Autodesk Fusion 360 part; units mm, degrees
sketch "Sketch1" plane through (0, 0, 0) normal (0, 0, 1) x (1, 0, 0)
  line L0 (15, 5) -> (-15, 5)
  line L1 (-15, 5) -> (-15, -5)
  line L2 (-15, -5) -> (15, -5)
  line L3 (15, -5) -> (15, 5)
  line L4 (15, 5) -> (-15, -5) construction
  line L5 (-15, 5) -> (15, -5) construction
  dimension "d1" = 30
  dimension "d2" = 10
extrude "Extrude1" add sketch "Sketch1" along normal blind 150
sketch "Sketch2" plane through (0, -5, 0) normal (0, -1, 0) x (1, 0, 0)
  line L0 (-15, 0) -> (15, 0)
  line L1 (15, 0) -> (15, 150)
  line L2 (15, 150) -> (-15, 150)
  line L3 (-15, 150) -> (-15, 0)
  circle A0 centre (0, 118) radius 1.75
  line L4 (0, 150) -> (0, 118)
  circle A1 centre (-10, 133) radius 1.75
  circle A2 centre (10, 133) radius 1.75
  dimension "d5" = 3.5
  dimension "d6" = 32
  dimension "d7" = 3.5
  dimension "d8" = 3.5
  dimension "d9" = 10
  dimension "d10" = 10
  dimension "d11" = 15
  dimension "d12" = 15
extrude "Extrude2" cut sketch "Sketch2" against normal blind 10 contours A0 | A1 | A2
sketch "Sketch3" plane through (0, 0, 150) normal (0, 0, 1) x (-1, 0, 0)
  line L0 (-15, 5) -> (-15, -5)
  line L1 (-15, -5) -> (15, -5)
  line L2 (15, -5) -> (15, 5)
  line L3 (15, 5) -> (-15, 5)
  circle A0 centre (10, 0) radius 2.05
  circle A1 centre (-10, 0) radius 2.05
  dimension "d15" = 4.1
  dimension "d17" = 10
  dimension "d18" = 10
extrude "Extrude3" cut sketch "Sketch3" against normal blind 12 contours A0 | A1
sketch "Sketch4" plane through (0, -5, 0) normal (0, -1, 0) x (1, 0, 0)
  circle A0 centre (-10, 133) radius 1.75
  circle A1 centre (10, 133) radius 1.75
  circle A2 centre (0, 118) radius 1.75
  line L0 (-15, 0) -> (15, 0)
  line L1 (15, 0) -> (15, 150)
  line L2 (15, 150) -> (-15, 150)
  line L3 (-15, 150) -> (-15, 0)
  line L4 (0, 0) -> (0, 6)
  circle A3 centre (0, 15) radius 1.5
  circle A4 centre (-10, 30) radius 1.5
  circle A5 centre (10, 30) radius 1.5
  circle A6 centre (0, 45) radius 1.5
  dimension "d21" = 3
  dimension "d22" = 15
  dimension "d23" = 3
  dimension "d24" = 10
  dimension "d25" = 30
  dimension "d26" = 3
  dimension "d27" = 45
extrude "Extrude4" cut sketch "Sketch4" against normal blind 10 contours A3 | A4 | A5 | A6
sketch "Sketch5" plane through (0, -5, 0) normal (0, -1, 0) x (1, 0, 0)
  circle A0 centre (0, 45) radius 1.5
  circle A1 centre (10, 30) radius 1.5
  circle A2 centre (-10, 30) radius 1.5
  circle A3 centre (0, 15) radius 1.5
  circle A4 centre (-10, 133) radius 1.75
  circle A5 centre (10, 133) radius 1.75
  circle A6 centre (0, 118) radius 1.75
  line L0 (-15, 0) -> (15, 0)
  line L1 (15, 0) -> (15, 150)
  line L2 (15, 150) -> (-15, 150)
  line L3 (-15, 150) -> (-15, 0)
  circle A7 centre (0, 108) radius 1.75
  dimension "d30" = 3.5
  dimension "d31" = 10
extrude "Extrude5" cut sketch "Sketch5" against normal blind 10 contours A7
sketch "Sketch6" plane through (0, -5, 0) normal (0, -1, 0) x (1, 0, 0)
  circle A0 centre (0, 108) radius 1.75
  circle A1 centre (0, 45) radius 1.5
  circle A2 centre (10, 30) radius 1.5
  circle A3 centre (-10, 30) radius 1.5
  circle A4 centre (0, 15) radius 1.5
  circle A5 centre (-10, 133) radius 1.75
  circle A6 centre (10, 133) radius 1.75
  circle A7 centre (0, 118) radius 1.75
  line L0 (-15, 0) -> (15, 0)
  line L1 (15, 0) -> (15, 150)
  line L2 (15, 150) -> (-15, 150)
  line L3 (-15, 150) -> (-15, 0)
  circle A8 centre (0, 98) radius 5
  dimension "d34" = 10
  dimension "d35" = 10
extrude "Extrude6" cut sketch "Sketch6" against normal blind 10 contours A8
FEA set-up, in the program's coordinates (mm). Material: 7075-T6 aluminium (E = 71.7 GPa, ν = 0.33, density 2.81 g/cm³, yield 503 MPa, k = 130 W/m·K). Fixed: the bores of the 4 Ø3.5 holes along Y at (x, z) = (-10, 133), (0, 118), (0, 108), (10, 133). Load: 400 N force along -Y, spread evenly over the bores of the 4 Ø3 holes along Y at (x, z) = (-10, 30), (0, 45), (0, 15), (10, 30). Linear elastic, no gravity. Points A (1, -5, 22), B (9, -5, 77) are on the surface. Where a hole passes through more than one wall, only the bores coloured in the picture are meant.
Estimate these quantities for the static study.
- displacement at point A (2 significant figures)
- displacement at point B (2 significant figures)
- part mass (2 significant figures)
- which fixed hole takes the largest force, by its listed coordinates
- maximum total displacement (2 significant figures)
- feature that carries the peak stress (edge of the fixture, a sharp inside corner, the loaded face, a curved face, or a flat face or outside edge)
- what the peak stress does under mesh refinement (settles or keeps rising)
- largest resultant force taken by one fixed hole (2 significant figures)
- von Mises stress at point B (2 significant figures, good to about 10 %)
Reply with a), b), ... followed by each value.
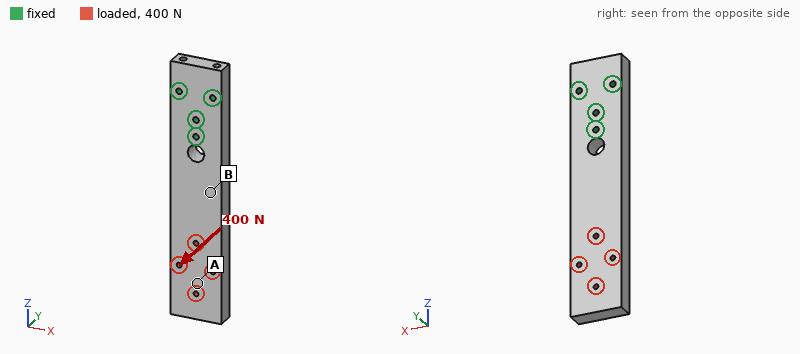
a) 0.55 mm
b) 0.12 mm
c) 120 g
d) (0, 108)
e) 0.74 mm
f) edge of the fixture
g) keeps rising
h) 1.6 kN
i) 38 MPa
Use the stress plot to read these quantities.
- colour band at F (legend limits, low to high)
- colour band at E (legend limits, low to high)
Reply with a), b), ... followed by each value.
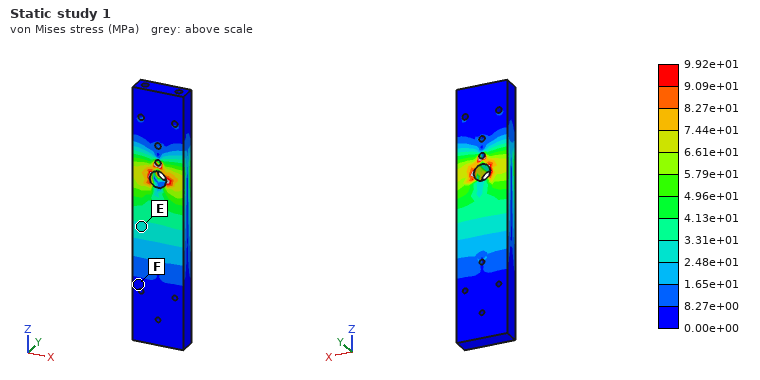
a) 0.00e+00 to 8.27e+00 MPa
b) 2.48e+01 to 3.31e+01 MPa
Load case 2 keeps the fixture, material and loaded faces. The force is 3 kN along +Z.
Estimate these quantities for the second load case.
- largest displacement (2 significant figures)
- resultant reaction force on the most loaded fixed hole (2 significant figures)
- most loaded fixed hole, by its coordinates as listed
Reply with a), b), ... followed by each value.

a) 15 µm
b) 1.3 kN
c) (0, 108)
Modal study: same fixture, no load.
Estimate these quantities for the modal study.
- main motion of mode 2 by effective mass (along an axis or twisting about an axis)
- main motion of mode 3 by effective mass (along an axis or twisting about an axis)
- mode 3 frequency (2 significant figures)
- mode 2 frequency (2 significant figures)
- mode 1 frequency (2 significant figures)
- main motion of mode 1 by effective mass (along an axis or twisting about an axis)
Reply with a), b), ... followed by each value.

a) along X
b) twisting about Z
c) 3800 Hz
d) 1600 Hz
e) 610 Hz
f) along Y
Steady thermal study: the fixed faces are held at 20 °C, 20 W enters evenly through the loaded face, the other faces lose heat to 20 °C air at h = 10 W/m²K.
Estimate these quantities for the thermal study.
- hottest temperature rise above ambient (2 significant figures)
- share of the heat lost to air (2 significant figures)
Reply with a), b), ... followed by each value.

a) 42 K
b) 12 %
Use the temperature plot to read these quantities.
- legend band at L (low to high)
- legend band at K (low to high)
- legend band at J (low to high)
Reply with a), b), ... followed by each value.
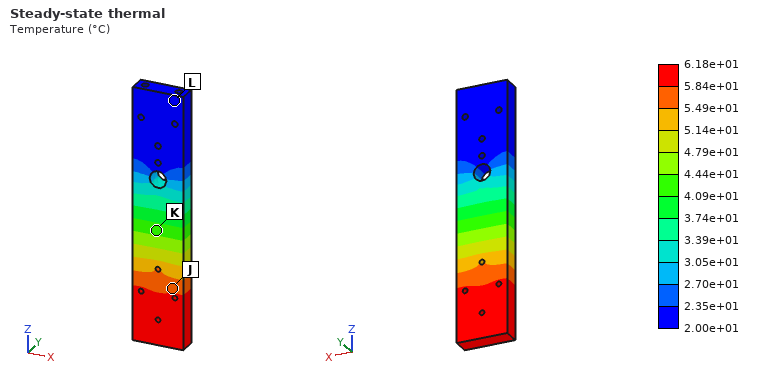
a) 2.00e+01 to 2.35e+01 °C
b) 4.09e+01 to 4.44e+01 °C
c) 5.49e+01 to 5.84e+01 °C
